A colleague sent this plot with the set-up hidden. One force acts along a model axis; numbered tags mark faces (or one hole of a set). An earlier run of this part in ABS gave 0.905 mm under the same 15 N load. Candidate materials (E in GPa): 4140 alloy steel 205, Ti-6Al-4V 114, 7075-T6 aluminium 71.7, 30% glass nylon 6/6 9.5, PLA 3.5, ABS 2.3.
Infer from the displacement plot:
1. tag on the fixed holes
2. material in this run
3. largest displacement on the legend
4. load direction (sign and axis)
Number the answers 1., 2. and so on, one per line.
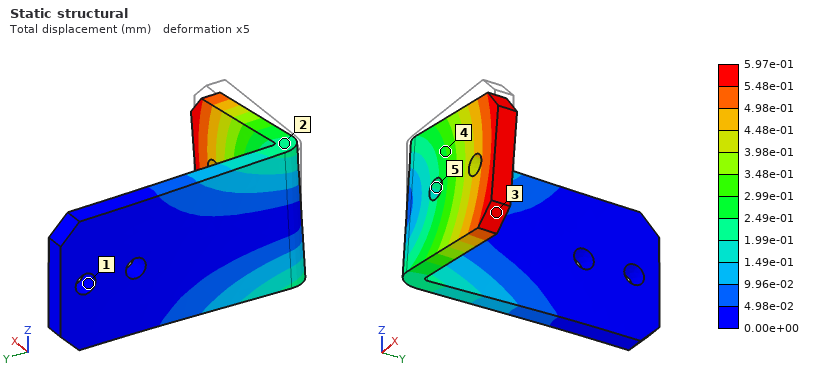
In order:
1. 1
2. PLA
3. 5.97e-01 mm
4. -Z
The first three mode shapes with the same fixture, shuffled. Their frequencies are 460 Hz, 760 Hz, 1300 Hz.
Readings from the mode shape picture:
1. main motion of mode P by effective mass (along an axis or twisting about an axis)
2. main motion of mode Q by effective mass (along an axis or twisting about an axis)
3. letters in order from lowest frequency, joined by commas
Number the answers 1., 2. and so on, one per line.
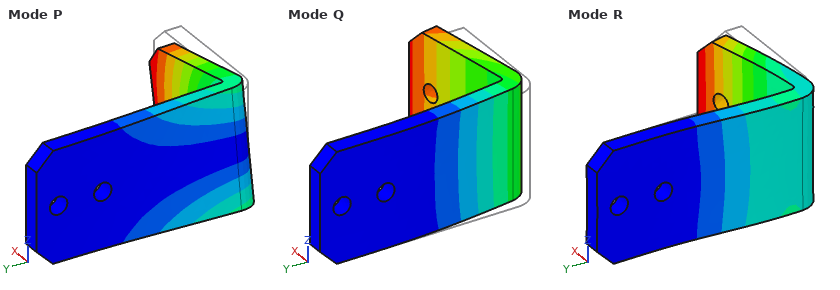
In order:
1. along Z
2. along X
3. Q, P, R
